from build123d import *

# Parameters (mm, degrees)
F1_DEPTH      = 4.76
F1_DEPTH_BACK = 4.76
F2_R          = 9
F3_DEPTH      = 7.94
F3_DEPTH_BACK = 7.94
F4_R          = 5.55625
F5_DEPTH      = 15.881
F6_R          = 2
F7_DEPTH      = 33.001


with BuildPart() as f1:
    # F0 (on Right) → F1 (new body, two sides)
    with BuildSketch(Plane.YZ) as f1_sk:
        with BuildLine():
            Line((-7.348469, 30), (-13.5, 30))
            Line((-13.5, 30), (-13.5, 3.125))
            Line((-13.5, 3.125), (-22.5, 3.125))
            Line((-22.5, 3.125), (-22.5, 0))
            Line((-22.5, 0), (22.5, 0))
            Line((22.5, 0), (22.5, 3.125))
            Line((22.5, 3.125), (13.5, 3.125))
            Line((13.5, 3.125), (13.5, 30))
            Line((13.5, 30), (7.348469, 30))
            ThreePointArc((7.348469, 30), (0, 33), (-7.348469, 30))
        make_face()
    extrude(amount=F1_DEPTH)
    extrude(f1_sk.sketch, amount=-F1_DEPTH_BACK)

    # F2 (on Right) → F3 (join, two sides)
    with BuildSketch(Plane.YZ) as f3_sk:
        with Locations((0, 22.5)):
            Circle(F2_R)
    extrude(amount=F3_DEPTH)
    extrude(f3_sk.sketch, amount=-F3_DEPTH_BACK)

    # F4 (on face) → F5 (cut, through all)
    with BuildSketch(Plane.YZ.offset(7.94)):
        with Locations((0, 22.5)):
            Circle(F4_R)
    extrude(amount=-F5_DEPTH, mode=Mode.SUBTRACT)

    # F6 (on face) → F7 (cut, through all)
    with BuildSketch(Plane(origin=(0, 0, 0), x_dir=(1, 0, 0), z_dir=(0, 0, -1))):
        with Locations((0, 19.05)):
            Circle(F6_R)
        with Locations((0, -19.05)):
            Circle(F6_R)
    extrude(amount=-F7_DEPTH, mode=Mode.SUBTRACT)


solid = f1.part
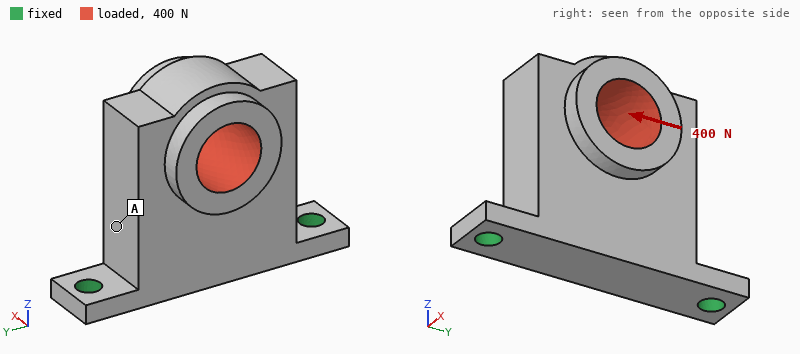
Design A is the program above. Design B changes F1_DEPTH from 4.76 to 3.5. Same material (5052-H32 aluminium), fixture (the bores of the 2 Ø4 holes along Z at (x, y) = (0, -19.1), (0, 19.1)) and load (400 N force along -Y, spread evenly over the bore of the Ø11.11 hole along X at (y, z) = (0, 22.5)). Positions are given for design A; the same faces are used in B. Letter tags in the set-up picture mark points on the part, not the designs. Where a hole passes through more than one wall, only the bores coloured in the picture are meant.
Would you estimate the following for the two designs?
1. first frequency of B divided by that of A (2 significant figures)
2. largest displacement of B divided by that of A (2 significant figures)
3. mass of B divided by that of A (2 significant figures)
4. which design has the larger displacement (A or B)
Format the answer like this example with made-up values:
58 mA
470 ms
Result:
0.92
1.1
0.91
B
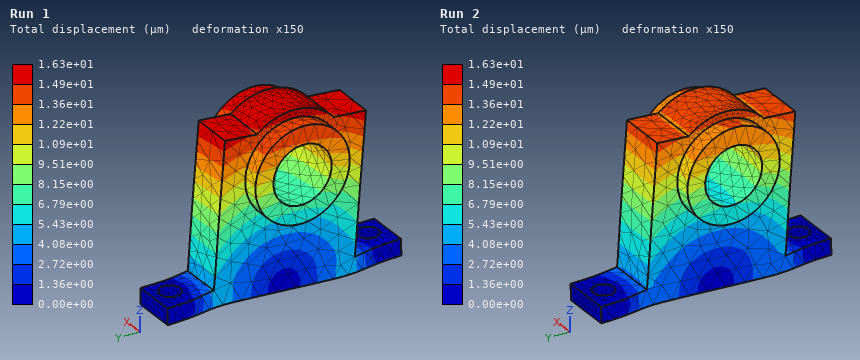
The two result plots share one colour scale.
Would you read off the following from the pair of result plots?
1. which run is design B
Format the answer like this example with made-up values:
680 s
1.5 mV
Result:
Run 1
